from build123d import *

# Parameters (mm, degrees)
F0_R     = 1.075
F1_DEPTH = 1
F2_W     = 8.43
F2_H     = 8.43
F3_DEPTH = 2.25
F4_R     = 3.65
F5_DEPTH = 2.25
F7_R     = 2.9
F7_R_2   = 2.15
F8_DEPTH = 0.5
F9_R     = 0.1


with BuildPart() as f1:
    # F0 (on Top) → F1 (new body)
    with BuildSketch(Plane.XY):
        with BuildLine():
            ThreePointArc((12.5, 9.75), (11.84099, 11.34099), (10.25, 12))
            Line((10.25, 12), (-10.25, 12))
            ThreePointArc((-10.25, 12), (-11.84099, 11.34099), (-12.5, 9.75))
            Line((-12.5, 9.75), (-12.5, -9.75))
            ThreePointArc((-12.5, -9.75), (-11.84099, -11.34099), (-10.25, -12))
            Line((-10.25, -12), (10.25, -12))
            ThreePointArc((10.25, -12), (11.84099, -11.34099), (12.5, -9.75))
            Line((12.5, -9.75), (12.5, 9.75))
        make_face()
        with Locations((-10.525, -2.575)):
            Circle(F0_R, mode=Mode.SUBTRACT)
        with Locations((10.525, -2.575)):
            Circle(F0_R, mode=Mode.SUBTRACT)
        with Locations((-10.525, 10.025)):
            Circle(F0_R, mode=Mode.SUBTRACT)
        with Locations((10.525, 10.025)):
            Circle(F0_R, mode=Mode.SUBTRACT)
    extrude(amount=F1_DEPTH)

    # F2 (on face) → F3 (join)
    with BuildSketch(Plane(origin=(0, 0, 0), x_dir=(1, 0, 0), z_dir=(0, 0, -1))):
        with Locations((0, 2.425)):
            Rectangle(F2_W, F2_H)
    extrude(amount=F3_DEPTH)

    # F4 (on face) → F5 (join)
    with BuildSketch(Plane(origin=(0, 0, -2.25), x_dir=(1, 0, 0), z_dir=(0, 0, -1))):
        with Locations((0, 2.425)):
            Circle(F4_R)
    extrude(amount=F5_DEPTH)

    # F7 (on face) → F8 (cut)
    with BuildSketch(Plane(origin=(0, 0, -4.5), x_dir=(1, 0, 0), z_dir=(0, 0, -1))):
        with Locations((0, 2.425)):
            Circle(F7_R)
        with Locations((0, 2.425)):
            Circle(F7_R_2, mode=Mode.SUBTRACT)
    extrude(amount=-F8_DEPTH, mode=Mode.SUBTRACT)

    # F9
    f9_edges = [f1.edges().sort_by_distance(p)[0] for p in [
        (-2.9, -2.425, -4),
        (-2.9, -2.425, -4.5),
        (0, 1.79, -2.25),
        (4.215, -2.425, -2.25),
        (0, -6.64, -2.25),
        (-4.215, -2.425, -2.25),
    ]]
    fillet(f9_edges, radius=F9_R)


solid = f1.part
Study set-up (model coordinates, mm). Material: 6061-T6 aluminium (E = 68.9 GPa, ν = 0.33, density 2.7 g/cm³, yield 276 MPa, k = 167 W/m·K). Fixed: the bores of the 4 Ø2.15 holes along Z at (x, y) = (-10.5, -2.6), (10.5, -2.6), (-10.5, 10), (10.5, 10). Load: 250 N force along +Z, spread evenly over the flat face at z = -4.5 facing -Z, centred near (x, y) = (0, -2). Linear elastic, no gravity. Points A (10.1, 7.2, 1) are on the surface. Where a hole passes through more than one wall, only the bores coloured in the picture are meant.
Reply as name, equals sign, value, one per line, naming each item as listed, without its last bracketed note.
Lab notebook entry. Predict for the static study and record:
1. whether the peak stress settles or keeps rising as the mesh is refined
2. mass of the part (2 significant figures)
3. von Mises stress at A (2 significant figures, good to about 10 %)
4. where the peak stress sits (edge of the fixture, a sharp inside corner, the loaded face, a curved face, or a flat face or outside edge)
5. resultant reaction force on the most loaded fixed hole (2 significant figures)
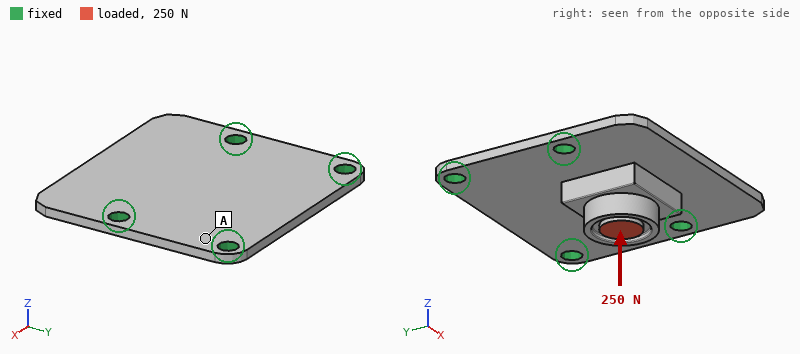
whether the peak stress settles or keeps rising as the mesh is refined = keeps rising
mass of the part = 2.2 g
von Mises stress at A = 34 MPa
where the peak stress sits = edge of the fixture
resultant reaction force on the most loaded fixed hole = 130 N
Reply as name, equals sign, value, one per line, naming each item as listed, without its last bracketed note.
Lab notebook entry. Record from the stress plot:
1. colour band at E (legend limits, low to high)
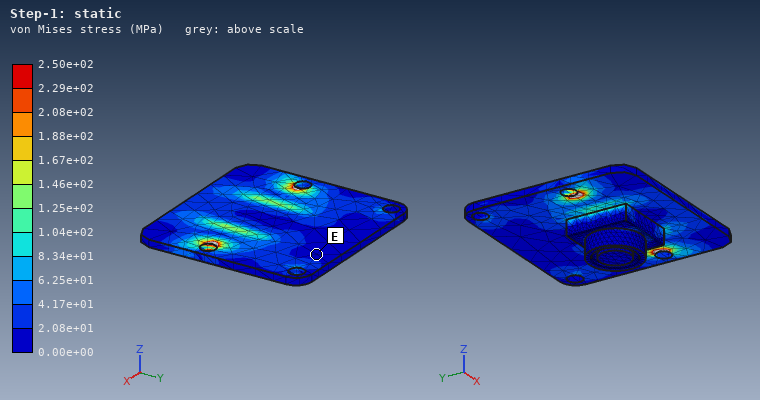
colour band at E = 0.00e+00 to 2.08e+01 MPa
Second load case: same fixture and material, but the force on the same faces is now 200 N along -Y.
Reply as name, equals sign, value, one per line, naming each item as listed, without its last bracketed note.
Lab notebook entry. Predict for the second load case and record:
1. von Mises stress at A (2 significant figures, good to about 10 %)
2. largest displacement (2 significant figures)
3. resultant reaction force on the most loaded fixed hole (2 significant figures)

von Mises stress at A = 47 MPa
largest displacement = 0.11 mm
resultant reaction force on the most loaded fixed hole = 68 N
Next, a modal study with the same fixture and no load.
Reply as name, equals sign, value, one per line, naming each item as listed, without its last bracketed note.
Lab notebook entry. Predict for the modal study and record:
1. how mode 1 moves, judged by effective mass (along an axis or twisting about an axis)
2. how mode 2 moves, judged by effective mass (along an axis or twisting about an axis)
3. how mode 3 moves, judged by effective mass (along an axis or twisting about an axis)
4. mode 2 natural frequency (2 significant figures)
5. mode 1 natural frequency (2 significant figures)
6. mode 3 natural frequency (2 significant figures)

how mode 1 moves, judged by effective mass = along Z
how mode 2 moves, judged by effective mass = along Z
how mode 3 moves, judged by effective mass = twisting about Y
mode 2 natural frequency = 11 kHz
mode 1 natural frequency = 8100 Hz
mode 3 natural frequency = 15 kHz
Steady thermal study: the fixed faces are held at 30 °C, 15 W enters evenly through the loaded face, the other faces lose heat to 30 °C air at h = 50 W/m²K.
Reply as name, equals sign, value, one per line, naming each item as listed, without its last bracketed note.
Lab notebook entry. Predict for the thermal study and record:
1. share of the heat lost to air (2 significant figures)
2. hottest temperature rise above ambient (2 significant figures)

share of the heat lost to air = 5.7 %
hottest temperature rise above ambient = 37 K
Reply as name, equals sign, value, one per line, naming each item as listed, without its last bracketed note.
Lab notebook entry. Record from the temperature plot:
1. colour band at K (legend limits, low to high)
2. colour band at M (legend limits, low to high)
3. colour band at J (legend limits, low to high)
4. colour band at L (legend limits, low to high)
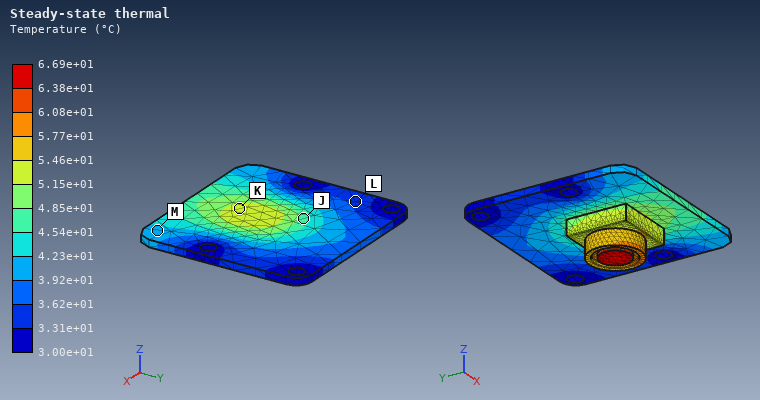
colour band at K = 5.15e+01 to 5.46e+01 °C
colour band at M = 3.92e+01 to 4.23e+01 °C
colour band at J = 4.54e+01 to 4.85e+01 °C
colour band at L = 3.31e+01 to 3.62e+01 °C
